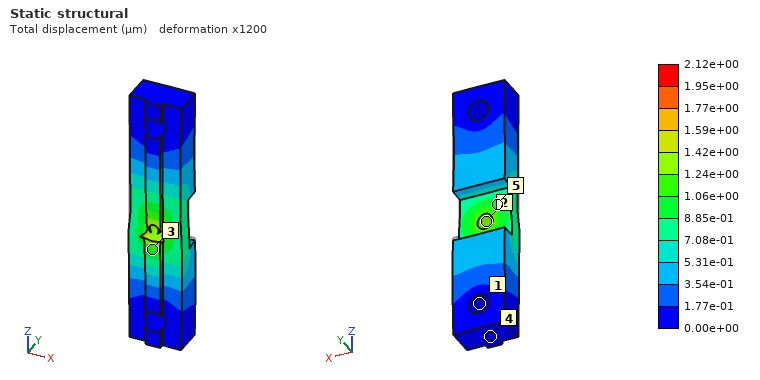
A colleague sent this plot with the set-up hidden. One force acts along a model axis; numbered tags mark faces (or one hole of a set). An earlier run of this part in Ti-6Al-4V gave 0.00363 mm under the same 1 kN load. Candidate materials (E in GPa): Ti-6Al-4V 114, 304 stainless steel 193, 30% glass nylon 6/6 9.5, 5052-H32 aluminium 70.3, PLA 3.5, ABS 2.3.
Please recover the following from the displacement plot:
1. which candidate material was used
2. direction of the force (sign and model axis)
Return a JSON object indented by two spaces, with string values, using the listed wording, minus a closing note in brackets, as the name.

{
  "which candidate material was used": "304 stainless steel",
  "direction of the force": "-Z"
}
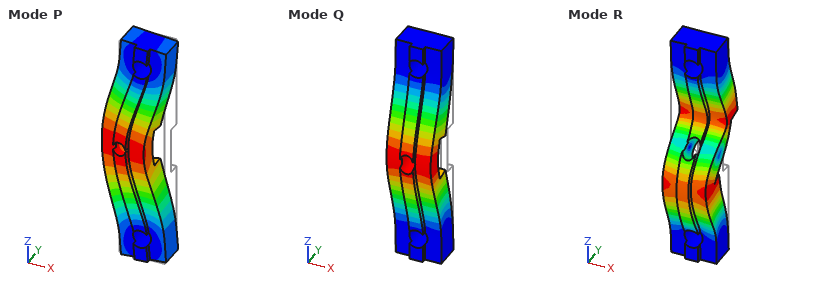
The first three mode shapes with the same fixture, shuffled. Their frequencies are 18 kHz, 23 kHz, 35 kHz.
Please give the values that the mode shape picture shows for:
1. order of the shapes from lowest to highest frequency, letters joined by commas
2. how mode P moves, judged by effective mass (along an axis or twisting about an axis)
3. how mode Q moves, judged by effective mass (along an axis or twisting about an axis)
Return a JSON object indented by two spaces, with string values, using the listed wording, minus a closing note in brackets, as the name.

{
  "order of the shapes from lowest to highest frequency, letters joined by commas": "Q, P, R",
  "how mode P moves, judged by effective mass": "along X",
  "how mode Q moves, judged by effective mass": "along Y"
}
